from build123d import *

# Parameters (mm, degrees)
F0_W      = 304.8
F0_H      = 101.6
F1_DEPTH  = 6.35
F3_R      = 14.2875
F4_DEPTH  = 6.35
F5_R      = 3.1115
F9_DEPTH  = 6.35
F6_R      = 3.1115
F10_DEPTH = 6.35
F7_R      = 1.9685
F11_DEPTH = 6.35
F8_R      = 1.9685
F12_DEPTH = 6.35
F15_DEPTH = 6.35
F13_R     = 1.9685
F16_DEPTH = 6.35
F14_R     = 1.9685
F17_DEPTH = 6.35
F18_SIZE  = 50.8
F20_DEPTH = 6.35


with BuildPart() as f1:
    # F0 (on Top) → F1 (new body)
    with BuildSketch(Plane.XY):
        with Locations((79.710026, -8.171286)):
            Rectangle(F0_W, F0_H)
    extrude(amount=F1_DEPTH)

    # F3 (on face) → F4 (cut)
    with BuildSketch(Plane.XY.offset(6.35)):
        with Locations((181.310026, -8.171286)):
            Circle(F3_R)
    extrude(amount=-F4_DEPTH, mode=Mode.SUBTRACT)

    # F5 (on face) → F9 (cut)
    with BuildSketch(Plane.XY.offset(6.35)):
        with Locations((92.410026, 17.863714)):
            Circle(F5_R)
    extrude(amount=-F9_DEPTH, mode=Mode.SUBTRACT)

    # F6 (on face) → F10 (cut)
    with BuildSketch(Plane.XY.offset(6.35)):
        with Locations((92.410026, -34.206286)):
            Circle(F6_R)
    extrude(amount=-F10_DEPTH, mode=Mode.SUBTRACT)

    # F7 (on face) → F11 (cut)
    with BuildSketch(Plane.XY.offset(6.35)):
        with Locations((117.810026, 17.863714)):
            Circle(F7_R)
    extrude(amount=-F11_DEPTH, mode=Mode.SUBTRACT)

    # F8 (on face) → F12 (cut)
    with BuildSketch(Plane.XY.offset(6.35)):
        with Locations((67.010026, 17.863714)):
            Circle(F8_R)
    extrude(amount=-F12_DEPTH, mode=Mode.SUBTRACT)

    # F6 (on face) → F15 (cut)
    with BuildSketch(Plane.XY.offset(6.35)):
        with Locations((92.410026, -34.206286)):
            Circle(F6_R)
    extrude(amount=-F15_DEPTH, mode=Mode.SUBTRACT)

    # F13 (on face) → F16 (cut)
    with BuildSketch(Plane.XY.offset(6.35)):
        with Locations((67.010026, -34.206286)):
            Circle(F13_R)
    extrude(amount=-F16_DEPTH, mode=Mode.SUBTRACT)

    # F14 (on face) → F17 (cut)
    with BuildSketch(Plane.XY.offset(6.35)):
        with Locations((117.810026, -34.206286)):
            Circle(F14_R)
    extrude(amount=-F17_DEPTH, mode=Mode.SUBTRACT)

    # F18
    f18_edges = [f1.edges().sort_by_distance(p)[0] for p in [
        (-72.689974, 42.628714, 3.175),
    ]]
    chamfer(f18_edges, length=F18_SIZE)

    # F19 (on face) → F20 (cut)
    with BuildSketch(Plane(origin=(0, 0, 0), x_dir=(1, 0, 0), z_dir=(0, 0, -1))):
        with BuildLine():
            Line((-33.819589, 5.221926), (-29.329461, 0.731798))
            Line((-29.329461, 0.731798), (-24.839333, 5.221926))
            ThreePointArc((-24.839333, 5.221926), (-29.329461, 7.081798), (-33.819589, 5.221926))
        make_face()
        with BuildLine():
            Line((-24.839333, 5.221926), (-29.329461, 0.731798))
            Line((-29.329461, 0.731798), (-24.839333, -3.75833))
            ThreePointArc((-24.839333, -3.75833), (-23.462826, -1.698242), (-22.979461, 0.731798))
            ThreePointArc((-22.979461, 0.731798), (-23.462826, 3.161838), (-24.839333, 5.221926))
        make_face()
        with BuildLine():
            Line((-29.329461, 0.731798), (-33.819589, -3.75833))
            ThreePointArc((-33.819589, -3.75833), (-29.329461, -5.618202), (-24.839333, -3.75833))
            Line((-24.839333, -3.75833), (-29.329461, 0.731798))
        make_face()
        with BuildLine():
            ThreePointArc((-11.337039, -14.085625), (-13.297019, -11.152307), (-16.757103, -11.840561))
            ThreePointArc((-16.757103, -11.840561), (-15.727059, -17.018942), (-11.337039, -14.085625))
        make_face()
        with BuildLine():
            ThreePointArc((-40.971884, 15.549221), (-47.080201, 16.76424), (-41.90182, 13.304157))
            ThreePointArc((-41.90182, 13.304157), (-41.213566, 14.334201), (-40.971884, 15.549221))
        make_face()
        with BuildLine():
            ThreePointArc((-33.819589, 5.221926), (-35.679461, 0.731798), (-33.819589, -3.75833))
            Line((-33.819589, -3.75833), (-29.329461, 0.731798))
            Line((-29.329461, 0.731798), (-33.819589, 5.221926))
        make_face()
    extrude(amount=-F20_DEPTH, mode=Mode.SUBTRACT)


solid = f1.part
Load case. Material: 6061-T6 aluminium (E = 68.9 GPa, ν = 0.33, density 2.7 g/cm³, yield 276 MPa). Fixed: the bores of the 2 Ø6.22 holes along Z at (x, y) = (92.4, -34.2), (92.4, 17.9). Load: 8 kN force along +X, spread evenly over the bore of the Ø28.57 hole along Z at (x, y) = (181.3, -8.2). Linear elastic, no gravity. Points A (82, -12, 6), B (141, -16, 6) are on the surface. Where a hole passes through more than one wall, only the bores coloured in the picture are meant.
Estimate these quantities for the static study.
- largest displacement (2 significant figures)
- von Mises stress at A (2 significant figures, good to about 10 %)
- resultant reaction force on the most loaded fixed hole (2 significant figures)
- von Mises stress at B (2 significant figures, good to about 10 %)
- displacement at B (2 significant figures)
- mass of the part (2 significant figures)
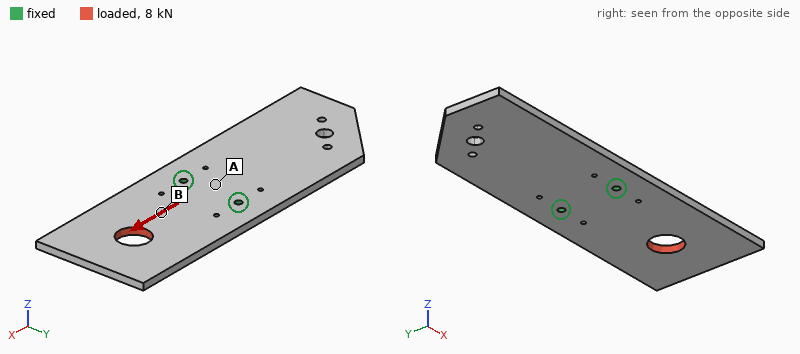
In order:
29 µm
4.6 MPa
4.0 kN
15 MPa
12 µm
490 g
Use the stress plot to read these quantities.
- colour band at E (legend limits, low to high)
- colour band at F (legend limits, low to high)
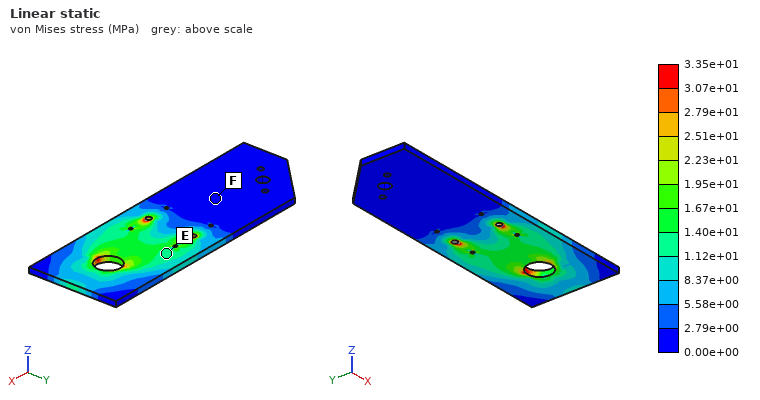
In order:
1.12e+01 to 1.40e+01 MPa
0.00e+00 to 2.79e+00 MPa
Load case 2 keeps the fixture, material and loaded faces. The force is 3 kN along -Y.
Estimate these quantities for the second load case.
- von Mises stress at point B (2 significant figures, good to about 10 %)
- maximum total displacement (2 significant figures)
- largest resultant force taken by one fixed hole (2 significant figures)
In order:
14 MPa
91 µm
5.1 kN
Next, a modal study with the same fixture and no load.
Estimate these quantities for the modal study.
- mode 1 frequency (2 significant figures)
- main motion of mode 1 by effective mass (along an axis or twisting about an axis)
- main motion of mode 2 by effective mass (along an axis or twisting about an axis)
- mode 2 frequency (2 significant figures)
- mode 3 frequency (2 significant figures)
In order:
210 Hz
along Z
along Z
270 Hz
760 Hz
